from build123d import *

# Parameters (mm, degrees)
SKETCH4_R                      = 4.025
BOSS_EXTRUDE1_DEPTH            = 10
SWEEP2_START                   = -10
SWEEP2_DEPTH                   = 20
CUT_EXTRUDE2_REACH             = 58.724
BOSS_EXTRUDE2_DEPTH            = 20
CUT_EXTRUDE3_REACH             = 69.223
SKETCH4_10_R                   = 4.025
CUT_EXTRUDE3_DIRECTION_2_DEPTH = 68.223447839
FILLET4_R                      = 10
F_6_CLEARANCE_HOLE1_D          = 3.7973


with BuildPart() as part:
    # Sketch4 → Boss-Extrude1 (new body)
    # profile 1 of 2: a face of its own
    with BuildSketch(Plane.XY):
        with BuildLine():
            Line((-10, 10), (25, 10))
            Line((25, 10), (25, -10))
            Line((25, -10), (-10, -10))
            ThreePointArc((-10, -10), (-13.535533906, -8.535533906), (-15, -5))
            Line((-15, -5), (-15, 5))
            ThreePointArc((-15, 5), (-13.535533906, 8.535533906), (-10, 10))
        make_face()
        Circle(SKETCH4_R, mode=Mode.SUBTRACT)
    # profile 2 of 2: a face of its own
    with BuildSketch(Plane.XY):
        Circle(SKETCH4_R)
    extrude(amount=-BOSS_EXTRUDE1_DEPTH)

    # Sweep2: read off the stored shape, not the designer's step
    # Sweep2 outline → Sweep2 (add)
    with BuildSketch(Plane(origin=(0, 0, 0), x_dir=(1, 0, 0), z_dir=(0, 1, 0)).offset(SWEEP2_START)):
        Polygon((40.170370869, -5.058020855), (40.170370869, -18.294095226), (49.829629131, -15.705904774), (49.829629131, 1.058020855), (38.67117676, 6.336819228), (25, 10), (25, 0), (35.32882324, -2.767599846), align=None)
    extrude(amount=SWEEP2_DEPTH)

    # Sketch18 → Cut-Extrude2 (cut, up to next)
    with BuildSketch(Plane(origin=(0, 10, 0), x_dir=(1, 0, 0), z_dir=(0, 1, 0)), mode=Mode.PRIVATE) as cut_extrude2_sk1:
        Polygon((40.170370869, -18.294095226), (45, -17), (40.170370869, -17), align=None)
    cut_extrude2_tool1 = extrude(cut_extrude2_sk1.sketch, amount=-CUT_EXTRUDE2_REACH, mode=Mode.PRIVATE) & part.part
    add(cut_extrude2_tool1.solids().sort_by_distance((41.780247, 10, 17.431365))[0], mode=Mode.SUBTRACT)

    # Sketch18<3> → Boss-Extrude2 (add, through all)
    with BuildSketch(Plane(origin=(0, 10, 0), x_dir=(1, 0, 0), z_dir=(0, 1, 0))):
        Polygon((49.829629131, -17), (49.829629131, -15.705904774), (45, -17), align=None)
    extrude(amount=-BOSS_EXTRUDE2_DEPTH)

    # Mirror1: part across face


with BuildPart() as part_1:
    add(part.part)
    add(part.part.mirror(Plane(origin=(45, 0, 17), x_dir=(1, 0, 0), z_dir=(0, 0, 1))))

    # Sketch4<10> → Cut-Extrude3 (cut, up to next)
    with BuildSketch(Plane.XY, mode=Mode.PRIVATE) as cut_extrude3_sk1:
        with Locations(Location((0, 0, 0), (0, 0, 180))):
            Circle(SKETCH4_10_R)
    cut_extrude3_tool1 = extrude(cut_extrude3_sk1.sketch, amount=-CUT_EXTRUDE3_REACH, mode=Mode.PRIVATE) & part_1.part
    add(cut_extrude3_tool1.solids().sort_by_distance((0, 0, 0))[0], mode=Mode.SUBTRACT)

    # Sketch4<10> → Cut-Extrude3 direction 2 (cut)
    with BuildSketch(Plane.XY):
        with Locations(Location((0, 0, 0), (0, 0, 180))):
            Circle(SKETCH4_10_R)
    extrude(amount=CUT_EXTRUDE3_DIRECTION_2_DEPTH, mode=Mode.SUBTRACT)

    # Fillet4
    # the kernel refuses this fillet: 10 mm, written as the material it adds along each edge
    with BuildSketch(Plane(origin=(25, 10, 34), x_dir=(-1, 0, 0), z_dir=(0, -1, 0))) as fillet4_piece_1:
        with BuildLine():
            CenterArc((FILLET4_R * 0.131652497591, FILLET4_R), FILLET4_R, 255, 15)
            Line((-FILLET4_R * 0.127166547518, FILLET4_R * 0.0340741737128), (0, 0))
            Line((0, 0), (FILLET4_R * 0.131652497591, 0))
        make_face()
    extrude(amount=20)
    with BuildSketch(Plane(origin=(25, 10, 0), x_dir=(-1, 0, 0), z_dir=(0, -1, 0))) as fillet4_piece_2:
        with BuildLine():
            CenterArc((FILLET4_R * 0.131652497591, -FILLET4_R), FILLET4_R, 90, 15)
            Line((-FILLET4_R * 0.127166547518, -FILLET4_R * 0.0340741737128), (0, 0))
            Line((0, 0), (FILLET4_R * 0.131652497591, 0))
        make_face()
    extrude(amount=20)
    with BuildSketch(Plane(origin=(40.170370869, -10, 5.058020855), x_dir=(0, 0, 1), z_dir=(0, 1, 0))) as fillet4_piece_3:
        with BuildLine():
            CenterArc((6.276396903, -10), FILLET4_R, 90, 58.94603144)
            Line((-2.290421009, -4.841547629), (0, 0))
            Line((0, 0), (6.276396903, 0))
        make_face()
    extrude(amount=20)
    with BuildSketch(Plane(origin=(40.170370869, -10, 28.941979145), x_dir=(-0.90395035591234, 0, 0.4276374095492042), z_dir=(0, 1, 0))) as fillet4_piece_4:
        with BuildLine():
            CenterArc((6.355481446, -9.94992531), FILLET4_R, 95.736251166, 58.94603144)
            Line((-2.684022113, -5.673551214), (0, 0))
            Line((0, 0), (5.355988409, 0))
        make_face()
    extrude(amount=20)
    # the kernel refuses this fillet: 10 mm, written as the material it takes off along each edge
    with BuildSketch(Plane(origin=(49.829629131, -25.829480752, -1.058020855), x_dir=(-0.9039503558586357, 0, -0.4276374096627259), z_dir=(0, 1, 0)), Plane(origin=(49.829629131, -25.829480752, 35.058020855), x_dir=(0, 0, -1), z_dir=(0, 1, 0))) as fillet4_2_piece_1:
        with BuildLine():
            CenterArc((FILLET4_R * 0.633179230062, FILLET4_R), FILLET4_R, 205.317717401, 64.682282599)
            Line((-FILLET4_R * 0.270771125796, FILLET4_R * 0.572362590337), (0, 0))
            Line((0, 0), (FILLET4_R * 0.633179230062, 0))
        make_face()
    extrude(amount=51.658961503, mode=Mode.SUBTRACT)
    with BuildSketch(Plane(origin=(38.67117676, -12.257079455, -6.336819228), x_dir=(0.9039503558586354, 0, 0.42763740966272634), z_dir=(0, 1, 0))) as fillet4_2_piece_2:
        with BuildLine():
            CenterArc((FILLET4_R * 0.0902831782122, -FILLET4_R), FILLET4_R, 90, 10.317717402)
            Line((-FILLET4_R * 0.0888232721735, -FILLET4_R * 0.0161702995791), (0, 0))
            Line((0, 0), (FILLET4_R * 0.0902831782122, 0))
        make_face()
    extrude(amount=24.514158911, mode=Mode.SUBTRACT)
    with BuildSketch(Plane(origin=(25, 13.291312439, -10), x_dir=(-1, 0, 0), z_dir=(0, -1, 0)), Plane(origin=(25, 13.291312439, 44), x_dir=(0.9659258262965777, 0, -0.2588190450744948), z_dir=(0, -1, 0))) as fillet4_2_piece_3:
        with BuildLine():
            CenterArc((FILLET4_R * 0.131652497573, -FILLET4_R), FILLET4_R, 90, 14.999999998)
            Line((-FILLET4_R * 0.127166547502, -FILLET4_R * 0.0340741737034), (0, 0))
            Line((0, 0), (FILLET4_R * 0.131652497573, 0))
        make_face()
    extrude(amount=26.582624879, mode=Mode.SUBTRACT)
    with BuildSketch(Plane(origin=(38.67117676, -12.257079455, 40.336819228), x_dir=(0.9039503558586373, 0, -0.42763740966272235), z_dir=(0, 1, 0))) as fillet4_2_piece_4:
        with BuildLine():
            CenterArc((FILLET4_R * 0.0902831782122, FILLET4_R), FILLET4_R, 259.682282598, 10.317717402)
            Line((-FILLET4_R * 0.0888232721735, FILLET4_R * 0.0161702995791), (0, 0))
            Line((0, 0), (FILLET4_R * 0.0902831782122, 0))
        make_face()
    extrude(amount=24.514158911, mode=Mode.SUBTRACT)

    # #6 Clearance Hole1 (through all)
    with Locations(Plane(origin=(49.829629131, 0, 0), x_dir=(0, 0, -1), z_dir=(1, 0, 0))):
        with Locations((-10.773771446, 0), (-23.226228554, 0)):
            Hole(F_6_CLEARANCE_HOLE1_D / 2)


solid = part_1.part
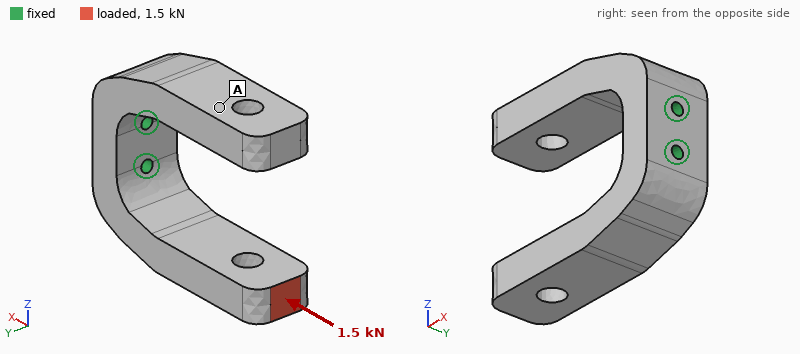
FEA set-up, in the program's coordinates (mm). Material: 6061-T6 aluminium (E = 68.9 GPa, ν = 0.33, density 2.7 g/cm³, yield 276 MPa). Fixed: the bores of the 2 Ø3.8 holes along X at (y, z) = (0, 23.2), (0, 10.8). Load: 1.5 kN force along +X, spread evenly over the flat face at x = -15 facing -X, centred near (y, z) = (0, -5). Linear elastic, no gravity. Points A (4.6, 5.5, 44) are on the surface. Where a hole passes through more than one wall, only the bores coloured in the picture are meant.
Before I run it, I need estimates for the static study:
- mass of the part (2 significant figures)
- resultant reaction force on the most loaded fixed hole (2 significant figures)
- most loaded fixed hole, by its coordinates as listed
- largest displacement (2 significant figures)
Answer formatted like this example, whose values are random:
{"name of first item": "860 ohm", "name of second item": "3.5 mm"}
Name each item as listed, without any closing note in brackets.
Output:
{"mass of the part": "77 g", "resultant reaction force on the most loaded fixed hole": "1.9 kN", "most loaded fixed hole, by its coordinates as listed": "(0, 10.8)", "largest displacement": "0.14 mm"}
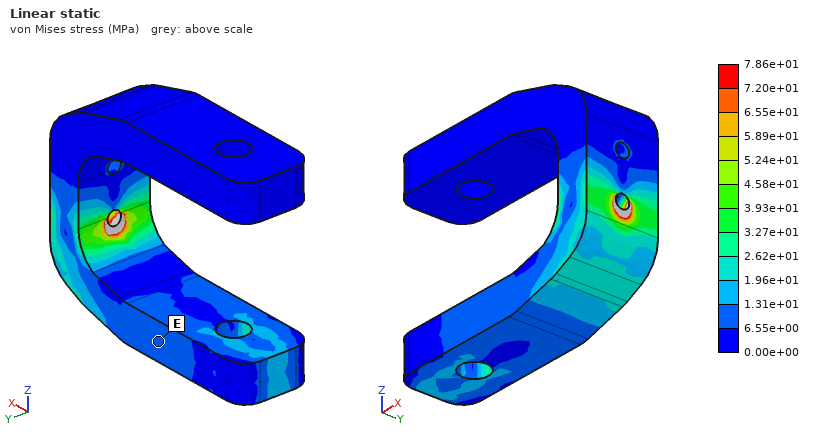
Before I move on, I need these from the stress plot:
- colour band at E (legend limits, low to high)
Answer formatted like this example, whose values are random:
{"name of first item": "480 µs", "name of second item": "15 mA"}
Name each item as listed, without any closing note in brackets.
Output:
{"colour band at E": "6.55e+00 to 1.31e+01 MPa"}
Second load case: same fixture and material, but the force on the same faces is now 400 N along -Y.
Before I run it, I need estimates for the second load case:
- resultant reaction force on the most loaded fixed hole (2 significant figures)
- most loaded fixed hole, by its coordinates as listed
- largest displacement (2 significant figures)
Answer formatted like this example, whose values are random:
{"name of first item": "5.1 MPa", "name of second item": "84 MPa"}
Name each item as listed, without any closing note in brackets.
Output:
{"resultant reaction force on the most loaded fixed hole": "730 N", "most loaded fixed hole, by its coordinates as listed": "(0, 10.8)", "largest displacement": "0.19 mm"}
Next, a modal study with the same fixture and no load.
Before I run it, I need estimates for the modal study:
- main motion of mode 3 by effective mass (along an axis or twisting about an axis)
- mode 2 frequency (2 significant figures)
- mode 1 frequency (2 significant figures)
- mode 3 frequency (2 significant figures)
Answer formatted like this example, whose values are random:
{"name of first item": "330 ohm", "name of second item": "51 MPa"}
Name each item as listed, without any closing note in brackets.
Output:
{"main motion of mode 3 by effective mass": "along Y", "mode 2 frequency": "1900 Hz", "mode 1 frequency": "1900 Hz", "mode 3 frequency": "2500 Hz"}
